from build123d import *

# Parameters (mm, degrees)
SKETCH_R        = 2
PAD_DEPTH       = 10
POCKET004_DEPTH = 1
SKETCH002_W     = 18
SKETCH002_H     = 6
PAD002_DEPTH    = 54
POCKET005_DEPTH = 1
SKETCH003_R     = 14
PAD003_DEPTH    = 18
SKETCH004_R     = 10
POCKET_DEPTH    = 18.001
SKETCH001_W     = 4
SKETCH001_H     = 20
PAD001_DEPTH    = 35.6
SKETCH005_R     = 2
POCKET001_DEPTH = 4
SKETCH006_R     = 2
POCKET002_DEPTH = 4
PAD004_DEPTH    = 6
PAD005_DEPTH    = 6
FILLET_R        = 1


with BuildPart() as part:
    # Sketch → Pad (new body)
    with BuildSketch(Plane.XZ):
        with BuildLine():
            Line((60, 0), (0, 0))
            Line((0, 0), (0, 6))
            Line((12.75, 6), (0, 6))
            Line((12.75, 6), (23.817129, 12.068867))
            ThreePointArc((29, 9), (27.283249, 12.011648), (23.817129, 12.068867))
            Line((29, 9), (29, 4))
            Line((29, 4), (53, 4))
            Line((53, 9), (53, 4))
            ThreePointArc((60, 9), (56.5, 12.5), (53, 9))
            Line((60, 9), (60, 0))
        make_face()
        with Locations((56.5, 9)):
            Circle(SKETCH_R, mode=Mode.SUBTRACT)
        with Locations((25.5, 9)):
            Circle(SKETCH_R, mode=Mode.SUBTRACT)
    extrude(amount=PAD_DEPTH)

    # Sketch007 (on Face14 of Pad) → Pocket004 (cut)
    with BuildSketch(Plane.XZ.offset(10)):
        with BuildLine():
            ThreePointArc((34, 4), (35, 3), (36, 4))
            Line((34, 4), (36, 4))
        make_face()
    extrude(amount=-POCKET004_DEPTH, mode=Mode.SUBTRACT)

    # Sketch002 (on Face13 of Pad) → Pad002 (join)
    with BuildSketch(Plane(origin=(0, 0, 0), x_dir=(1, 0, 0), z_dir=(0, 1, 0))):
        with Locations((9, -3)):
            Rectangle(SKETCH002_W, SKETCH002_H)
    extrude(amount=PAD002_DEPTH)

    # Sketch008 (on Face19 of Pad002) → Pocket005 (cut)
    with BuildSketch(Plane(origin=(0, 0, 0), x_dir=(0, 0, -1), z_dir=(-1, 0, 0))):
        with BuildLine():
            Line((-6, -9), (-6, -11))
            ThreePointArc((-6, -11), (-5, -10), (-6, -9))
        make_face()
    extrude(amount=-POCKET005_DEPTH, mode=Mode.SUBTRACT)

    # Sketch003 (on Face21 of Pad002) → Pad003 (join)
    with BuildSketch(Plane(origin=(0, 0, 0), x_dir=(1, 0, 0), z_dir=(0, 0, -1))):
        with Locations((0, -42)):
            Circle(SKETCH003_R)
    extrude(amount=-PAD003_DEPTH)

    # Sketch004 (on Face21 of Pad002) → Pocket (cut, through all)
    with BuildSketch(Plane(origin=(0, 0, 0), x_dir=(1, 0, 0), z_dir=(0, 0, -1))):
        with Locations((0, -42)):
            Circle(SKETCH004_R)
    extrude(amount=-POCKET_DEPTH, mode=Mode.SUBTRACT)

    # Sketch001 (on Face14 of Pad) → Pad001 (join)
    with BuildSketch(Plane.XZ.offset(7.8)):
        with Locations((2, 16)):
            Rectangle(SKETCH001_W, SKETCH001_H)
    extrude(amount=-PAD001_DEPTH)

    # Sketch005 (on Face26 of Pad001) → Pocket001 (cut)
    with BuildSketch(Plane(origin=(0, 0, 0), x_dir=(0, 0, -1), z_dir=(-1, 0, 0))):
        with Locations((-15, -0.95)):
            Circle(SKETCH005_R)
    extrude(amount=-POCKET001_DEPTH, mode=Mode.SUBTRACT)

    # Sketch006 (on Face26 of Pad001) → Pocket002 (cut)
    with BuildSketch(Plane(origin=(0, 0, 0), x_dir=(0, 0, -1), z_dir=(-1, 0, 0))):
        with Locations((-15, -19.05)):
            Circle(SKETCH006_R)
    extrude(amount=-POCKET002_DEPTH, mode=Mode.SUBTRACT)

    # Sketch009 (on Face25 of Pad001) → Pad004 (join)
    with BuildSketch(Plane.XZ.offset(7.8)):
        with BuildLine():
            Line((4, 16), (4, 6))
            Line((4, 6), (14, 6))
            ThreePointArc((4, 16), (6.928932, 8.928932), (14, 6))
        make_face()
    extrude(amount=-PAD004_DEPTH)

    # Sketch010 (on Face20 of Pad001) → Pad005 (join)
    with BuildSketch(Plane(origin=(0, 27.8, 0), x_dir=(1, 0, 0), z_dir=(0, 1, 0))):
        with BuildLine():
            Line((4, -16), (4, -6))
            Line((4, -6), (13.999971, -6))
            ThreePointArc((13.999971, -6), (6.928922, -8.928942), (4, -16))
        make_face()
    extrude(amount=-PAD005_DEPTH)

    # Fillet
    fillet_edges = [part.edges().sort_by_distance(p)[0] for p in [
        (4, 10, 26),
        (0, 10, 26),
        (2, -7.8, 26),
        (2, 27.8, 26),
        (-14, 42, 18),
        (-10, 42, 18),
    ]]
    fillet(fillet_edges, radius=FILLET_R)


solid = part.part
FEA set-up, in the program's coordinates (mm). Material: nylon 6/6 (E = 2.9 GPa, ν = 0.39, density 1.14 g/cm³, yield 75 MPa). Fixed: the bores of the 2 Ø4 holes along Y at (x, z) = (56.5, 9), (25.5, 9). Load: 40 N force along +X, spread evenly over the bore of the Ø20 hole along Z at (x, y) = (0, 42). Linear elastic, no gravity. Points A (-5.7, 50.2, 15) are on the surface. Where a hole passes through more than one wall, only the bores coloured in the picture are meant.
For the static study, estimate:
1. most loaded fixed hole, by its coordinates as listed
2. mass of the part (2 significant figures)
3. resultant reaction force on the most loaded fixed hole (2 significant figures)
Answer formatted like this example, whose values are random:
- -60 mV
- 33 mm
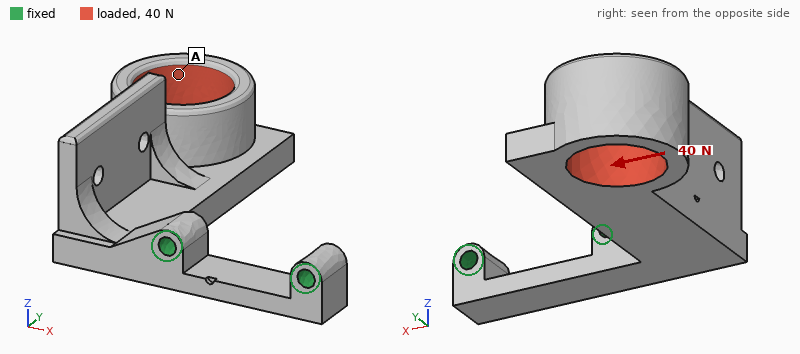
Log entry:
- (25.5, 9)
- 19 g
- 40 N
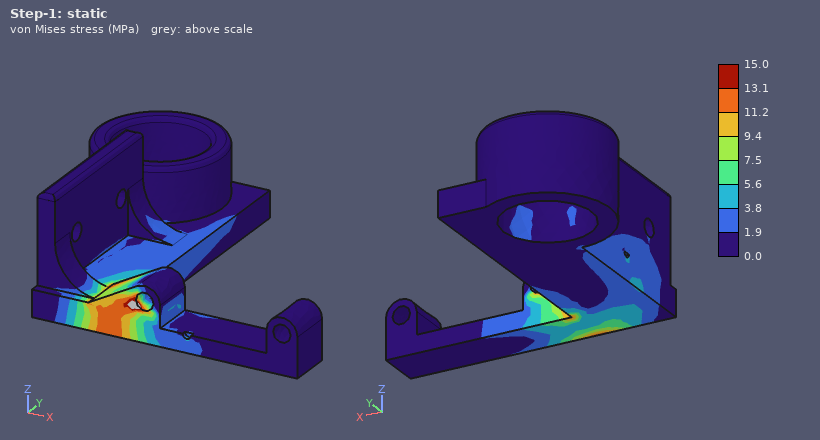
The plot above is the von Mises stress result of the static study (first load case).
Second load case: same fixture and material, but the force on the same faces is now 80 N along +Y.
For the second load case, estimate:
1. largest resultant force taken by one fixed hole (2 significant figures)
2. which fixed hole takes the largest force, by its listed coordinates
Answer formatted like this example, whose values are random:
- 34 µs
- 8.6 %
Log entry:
- 91 N
- (25.5, 9)
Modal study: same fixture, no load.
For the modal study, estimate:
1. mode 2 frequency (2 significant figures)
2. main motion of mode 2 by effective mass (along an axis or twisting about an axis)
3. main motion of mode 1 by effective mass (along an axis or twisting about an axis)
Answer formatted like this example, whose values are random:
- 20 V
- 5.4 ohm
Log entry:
- 360 Hz
- along X
- along Z
